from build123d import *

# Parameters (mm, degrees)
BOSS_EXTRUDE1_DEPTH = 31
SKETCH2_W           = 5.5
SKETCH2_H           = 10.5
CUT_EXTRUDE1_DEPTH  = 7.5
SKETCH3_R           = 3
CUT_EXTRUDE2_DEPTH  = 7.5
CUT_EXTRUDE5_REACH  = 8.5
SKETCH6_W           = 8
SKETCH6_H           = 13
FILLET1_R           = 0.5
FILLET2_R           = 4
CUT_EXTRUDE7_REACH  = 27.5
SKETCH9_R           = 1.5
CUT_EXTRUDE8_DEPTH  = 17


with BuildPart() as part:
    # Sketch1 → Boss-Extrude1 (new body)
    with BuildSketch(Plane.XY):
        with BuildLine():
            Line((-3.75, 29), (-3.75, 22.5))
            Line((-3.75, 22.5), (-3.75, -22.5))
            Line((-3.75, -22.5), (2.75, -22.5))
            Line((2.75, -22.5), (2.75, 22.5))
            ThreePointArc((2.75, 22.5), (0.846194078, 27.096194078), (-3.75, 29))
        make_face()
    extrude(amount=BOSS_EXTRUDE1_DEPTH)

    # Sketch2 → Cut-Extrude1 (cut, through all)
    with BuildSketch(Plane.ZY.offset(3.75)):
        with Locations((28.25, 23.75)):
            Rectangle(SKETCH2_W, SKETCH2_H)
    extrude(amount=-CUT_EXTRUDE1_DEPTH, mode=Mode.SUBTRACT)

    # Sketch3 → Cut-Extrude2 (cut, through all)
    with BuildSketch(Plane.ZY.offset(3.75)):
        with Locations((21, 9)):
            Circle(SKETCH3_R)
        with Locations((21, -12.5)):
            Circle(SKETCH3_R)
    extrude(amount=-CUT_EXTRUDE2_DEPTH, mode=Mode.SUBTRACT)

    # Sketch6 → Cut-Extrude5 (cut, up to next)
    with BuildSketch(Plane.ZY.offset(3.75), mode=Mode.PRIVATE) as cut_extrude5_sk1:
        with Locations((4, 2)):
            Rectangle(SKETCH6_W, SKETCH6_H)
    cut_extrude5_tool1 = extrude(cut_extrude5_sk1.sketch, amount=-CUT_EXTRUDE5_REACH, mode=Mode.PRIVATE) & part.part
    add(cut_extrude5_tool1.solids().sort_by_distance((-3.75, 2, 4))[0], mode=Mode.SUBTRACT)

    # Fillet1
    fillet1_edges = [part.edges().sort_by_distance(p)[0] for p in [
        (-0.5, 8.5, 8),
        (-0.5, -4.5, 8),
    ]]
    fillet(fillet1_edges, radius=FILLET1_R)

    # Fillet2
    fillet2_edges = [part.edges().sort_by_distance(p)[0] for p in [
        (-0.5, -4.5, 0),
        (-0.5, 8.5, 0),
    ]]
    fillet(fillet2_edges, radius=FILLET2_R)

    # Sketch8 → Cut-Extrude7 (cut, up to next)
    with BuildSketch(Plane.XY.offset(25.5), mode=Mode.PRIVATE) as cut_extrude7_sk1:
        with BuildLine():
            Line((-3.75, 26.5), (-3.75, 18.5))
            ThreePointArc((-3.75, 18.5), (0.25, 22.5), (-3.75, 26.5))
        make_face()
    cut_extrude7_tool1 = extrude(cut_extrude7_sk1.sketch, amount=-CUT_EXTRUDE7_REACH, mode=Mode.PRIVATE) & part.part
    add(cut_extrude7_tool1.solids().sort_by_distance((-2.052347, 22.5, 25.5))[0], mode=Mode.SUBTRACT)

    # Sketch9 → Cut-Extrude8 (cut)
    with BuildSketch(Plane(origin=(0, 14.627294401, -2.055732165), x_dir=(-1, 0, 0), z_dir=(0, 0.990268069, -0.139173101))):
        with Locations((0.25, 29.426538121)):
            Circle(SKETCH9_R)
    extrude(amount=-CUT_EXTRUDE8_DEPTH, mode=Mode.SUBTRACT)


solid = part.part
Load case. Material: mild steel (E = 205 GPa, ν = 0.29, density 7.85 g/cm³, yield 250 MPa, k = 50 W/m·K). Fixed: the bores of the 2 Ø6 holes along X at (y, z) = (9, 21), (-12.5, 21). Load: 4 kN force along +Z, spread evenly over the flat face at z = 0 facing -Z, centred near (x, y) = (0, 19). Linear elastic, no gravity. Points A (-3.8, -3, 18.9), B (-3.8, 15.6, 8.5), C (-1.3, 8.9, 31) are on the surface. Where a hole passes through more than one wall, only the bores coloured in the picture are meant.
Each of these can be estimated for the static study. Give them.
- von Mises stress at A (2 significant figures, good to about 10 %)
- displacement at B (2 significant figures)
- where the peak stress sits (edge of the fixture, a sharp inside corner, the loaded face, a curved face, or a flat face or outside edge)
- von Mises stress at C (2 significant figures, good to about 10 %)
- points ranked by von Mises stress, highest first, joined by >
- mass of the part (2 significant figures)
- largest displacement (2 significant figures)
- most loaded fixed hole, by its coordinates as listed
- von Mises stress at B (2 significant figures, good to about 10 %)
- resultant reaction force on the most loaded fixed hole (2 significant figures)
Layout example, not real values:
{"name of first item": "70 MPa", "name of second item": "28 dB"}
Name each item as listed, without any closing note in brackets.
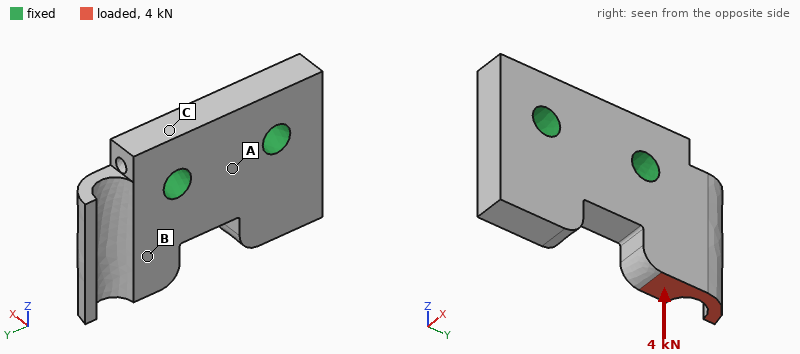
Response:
{"von Mises stress at A": "17 MPa", "displacement at B": "8.1 µm", "where the peak stress sits": "a curved face", "von Mises stress at C": "42 MPa", "points ranked by von Mises stress, highest first, joined by >": "B > C > A", "mass of the part": "62 g", "largest displacement": "25 µm", "most loaded fixed hole, by its coordinates as listed": "(9, 21)", "von Mises stress at B": "62 MPa", "resultant reaction force on the most loaded fixed hole": "5.1 kN"}
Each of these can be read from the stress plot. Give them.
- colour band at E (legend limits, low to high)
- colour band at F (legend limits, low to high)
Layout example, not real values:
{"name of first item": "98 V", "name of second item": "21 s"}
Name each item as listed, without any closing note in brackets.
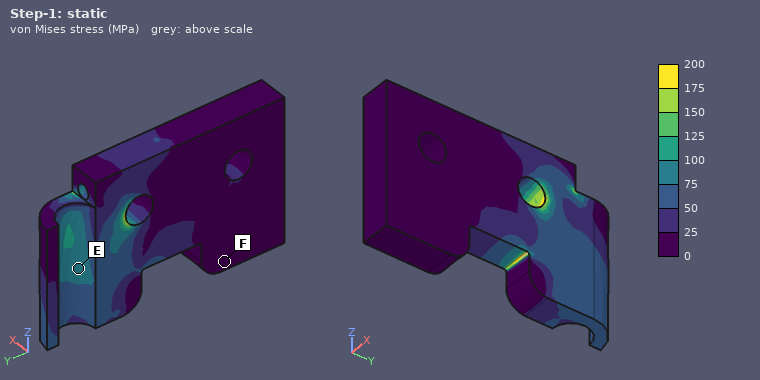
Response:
{"colour band at E": "75 to 100 MPa", "colour band at F": "0 to 25 MPa"}
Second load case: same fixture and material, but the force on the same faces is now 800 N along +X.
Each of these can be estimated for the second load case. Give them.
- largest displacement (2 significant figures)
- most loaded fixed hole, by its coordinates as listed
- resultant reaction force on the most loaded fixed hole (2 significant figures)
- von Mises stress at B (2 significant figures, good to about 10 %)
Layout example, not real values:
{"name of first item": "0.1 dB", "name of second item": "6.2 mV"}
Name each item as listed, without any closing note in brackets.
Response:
{"largest displacement": "63 µm", "most loaded fixed hole, by its coordinates as listed": "(9, 21)", "resultant reaction force on the most loaded fixed hole": "940 N", "von Mises stress at B": "76 MPa"}
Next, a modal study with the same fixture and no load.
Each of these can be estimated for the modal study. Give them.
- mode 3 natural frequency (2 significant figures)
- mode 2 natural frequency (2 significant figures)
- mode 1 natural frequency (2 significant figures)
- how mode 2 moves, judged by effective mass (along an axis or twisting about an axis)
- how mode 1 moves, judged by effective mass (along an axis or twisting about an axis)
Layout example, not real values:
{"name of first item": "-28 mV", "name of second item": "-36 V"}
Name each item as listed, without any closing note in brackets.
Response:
{"mode 3 natural frequency": "16 kHz", "mode 2 natural frequency": "14 kHz", "mode 1 natural frequency": "10 kHz", "how mode 2 moves, judged by effective mass": "along X", "how mode 1 moves, judged by effective mass": "along X"}
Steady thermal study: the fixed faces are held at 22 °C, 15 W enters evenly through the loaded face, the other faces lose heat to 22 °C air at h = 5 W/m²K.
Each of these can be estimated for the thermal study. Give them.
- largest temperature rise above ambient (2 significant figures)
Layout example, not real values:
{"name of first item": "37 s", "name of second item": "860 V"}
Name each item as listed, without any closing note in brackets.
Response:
{"largest temperature rise above ambient": "75 K"}
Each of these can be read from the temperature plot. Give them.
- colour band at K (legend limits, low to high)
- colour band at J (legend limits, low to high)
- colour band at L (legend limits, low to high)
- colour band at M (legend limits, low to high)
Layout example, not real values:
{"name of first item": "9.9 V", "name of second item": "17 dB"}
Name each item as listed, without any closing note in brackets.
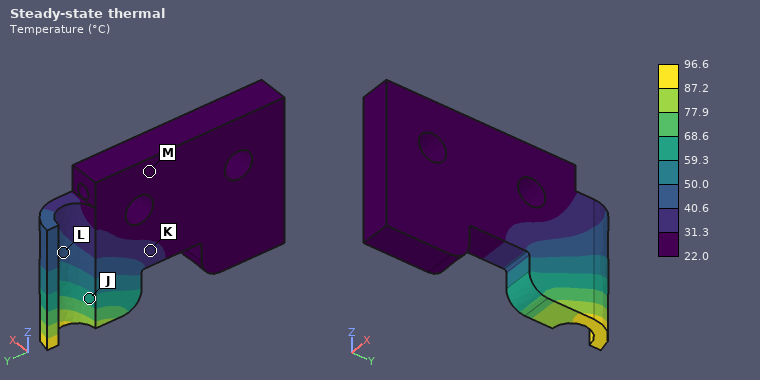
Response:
{"colour band at K": "31.3 to 40.6 °C", "colour band at J": "59.3 to 68.6 °C", "colour band at L": "40.6 to 50.0 °C", "colour band at M": "22.0 to 31.3 °C"}
